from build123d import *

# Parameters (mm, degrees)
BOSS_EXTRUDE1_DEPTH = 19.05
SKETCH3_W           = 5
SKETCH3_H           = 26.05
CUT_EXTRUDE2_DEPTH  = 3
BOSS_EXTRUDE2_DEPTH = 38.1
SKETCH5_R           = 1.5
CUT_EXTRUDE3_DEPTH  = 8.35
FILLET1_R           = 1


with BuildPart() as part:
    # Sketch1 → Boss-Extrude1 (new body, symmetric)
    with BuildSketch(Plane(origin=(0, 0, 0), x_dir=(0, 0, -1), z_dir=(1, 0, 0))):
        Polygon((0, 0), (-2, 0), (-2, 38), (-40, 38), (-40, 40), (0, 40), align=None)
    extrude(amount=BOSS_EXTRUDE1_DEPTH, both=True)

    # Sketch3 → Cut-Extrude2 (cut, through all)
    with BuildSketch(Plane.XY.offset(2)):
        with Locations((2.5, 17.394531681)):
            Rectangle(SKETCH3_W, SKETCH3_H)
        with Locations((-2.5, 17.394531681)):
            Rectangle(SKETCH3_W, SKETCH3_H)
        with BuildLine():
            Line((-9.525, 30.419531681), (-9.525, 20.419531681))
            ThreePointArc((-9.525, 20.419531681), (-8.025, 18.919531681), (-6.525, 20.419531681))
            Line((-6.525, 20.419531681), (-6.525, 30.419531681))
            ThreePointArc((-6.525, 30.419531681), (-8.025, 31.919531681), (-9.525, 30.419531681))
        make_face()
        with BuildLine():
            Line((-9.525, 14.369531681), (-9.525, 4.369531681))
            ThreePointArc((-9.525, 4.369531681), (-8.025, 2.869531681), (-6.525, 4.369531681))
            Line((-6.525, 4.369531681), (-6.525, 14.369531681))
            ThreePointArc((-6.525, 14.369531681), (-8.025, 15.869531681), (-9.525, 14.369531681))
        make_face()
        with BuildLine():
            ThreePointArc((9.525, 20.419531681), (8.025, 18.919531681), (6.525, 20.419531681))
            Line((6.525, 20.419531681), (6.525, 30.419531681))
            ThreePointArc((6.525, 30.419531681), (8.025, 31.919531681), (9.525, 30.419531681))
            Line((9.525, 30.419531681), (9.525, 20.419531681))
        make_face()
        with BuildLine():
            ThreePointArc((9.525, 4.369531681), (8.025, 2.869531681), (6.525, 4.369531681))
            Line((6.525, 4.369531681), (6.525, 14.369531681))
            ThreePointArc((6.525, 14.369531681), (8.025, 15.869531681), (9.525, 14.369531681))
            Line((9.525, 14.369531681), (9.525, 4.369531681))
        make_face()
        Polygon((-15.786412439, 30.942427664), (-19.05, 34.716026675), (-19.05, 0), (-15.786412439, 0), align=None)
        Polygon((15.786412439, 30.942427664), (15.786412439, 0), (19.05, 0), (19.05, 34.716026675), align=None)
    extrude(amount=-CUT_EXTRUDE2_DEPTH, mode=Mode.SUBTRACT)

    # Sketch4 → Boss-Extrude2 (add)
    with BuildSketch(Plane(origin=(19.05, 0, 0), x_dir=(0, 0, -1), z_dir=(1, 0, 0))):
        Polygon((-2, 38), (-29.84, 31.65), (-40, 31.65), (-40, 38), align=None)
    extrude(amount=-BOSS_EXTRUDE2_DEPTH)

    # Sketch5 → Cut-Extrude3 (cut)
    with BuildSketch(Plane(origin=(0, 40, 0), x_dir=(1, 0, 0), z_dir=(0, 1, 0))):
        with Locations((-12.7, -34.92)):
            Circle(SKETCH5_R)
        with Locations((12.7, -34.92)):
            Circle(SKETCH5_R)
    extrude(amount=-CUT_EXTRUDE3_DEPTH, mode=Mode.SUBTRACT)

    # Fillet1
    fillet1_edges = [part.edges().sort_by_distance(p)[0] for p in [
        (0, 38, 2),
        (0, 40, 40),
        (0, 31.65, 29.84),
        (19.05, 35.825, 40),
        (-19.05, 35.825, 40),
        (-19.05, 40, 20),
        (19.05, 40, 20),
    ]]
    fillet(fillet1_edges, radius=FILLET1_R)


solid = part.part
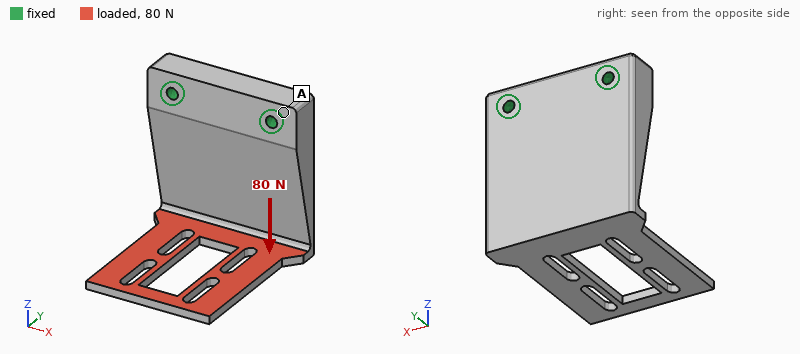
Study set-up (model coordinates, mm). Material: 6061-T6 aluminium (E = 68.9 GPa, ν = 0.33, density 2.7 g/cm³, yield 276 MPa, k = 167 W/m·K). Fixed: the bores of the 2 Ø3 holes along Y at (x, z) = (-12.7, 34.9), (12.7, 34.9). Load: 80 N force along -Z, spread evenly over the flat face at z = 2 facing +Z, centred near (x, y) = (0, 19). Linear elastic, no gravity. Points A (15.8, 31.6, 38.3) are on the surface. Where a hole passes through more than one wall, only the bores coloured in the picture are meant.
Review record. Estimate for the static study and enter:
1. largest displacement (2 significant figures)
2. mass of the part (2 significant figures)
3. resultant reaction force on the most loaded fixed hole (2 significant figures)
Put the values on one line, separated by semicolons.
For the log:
0.69 mm; 28 g; 40 N
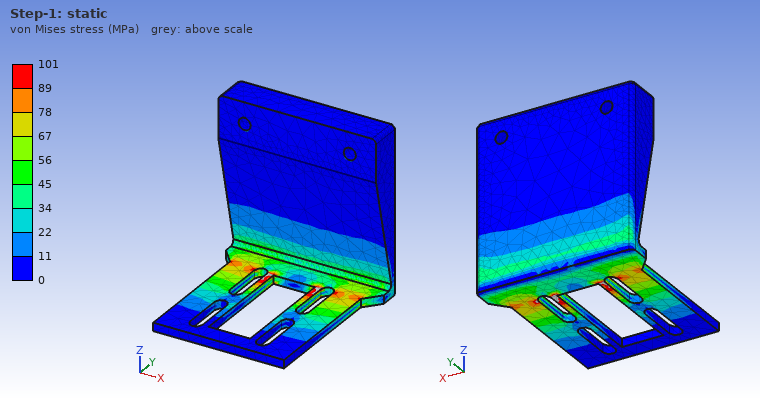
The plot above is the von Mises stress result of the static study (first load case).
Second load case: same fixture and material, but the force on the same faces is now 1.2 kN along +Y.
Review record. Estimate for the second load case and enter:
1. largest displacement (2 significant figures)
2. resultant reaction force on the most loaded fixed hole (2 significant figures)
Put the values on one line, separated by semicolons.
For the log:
0.33 mm; 600 N
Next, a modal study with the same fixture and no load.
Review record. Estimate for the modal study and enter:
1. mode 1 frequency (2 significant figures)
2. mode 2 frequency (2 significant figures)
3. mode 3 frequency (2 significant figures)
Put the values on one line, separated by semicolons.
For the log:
1000 Hz; 2300 Hz; 3100 Hz
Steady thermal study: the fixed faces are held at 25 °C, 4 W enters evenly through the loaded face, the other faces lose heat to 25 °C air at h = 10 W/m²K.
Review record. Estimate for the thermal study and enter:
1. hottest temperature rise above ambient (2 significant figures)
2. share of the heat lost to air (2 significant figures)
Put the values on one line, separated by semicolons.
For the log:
16 K; 5.5 %
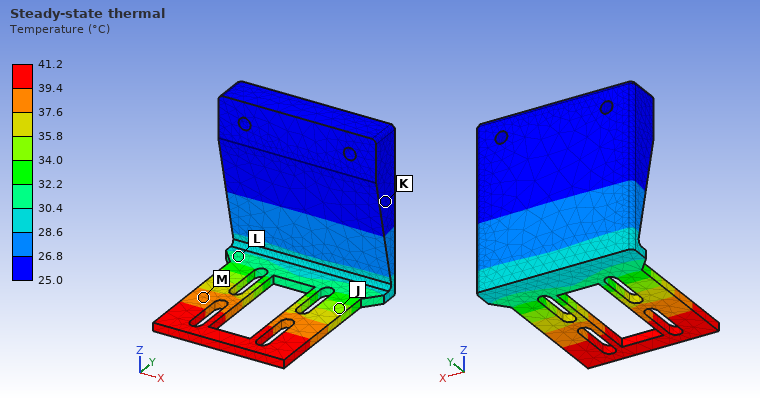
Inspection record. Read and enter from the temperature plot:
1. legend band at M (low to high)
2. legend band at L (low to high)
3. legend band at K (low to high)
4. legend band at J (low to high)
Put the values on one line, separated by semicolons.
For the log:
37.6 to 39.4 °C; 30.4 to 32.2 °C; 25.0 to 26.8 °C; 34.0 to 35.8 °C
